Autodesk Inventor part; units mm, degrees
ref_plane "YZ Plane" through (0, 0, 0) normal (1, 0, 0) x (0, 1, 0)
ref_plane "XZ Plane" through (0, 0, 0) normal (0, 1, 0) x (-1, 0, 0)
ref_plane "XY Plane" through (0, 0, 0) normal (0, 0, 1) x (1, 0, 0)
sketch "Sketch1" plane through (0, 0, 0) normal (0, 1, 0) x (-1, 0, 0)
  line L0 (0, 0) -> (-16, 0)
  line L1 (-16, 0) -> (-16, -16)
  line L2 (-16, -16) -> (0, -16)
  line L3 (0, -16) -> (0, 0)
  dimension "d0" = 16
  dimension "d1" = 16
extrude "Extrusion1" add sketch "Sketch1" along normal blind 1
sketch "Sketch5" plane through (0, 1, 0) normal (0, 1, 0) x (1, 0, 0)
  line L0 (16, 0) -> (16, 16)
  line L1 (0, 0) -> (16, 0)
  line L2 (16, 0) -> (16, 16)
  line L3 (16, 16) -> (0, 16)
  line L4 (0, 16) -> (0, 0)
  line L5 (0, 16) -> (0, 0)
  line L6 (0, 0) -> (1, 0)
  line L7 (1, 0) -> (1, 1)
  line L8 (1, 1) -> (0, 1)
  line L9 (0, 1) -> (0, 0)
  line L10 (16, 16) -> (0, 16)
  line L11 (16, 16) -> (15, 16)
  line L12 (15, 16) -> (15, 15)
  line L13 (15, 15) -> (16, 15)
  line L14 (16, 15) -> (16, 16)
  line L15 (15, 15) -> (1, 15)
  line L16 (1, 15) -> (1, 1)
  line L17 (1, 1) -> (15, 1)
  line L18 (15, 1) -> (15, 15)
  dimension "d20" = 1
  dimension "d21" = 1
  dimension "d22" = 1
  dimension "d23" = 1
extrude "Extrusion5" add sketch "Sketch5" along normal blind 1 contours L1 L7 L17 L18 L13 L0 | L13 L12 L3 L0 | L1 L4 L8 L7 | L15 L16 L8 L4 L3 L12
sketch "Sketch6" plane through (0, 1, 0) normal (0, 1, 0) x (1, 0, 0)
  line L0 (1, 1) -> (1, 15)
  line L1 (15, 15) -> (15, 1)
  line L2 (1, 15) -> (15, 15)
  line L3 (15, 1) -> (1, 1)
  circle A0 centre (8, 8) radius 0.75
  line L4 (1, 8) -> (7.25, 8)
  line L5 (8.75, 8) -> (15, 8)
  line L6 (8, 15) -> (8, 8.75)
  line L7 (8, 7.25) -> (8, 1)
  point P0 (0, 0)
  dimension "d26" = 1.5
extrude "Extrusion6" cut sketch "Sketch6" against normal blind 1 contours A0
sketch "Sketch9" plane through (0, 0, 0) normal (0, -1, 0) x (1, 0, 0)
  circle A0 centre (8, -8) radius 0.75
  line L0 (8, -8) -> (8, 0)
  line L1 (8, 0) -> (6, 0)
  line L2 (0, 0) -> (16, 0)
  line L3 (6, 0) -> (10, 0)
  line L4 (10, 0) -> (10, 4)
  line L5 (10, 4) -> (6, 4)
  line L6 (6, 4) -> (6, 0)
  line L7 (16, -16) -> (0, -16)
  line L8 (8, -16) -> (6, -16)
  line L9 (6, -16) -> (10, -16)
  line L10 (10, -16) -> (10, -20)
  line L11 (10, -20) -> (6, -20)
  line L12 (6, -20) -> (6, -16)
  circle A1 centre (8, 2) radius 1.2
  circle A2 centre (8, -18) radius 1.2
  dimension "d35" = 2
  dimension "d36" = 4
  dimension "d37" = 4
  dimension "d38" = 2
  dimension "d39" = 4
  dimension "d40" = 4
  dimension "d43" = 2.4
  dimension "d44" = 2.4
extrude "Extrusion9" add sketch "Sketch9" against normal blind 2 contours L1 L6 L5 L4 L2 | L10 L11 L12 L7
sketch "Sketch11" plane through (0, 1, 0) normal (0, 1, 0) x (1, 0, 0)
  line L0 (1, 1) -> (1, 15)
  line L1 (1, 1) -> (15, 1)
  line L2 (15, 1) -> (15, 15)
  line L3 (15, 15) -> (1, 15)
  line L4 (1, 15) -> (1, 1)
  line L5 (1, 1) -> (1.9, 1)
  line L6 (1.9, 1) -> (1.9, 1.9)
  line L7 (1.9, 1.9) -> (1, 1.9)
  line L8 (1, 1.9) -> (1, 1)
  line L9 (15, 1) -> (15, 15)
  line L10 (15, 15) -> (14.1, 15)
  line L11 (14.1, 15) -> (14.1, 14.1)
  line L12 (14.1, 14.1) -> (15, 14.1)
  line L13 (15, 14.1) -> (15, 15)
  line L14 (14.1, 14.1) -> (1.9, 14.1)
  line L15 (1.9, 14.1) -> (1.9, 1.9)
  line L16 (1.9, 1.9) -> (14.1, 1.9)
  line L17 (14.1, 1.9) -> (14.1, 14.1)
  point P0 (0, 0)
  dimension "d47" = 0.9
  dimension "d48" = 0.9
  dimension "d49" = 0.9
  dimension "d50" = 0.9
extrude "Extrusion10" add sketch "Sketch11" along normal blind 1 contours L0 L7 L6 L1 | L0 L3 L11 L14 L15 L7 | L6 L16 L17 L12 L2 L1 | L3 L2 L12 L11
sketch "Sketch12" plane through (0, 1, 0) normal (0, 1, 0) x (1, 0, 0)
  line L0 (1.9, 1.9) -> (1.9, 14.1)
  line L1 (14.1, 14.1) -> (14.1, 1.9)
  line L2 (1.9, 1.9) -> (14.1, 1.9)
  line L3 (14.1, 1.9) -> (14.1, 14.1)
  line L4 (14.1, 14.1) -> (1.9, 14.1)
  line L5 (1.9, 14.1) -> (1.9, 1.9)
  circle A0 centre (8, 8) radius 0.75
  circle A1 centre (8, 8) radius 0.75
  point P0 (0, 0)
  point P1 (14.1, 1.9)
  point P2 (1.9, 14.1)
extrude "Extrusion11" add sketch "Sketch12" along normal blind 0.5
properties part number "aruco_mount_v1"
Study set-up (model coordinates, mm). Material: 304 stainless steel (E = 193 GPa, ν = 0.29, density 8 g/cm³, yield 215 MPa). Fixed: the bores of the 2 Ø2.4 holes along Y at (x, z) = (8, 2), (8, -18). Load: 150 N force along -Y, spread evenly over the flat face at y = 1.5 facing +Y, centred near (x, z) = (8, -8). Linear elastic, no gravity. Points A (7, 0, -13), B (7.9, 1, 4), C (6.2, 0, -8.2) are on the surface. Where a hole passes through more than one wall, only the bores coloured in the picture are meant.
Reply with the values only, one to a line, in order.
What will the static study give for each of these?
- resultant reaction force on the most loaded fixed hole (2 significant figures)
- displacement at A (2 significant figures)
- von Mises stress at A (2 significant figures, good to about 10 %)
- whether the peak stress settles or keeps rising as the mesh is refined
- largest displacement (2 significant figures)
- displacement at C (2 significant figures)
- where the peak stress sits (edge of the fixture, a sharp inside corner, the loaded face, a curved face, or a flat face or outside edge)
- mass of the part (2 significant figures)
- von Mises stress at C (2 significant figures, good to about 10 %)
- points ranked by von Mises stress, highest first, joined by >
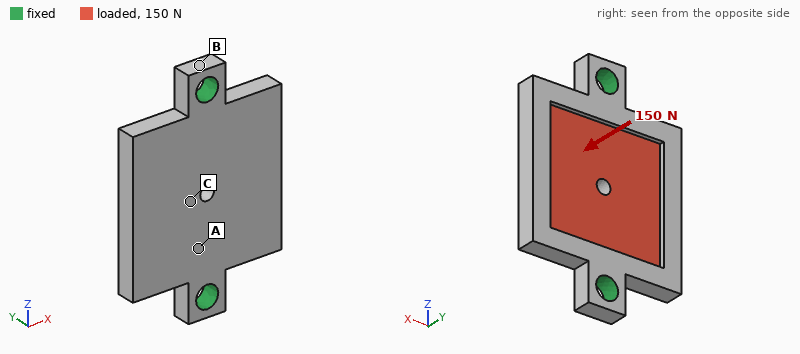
85 N
2.7 µm
19 MPa
keeps rising
6.6 µm
5.1 µm
edge of the fixture
3.8 g
34 MPa
C > A > B
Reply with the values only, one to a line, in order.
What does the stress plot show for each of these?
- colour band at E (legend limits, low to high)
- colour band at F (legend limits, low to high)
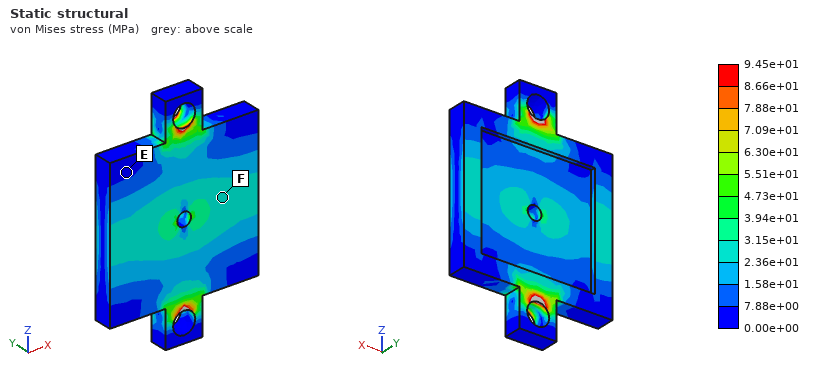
0.00e+00 to 7.88e+00 MPa
2.36e+01 to 3.15e+01 MPa
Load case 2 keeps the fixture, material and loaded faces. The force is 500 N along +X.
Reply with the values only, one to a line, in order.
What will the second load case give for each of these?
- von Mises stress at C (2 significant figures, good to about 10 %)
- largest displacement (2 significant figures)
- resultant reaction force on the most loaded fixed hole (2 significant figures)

9.4 MPa
6.8 µm
250 N
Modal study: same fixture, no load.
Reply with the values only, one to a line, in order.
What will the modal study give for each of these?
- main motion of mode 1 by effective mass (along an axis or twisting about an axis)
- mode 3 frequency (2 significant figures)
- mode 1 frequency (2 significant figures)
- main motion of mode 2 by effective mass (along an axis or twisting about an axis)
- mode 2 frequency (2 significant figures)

twisting about Z
27 kHz
11 kHz
along Y
15 kHz
